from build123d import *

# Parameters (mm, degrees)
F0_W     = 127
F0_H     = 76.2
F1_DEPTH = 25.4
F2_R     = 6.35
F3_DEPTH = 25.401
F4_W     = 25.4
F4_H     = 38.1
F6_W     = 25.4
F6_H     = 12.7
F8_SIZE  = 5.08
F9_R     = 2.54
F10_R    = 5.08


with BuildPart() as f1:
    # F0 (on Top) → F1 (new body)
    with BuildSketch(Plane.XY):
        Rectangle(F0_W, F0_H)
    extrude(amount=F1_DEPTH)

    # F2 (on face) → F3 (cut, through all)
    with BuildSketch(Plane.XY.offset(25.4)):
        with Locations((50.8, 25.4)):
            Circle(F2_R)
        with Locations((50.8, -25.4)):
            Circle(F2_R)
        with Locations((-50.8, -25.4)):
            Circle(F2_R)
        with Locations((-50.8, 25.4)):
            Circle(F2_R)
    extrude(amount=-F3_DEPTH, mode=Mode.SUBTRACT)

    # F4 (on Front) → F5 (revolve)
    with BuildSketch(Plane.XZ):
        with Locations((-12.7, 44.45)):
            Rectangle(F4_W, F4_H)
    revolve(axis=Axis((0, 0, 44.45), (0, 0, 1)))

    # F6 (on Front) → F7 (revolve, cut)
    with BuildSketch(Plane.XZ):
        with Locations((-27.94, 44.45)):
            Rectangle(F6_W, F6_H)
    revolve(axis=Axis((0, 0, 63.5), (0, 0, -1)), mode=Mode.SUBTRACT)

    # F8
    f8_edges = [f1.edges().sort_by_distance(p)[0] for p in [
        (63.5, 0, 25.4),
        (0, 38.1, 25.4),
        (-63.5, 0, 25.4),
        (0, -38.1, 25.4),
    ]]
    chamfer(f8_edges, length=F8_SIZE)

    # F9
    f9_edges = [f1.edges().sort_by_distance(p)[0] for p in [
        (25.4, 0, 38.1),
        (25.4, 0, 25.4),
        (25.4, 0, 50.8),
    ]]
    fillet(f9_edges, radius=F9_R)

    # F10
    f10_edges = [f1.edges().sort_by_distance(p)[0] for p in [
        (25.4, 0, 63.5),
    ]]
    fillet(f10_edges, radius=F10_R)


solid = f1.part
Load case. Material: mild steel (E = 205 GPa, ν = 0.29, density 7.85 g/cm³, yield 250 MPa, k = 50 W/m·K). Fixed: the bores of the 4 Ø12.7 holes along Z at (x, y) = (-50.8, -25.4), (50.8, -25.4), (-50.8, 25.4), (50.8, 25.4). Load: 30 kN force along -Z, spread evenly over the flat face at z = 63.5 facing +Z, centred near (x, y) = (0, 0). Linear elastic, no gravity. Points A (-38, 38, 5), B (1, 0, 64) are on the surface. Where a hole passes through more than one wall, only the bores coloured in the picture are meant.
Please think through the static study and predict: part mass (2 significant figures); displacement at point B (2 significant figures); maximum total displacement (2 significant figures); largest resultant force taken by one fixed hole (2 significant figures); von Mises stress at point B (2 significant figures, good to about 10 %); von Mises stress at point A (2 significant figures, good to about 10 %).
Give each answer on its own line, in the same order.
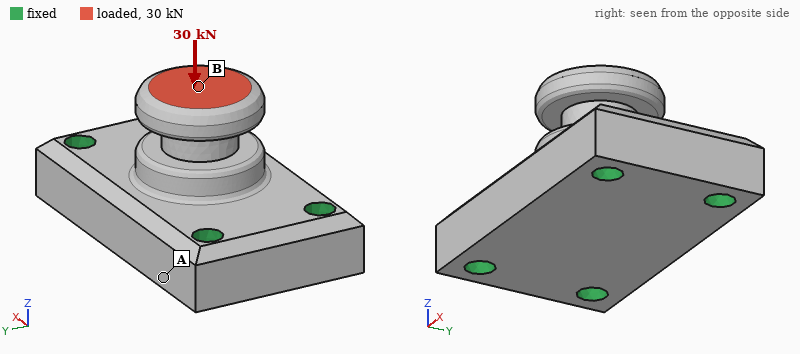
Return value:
2.3 kg
14 µm
15 µm
7.8 kN
39 MPa
11 MPa
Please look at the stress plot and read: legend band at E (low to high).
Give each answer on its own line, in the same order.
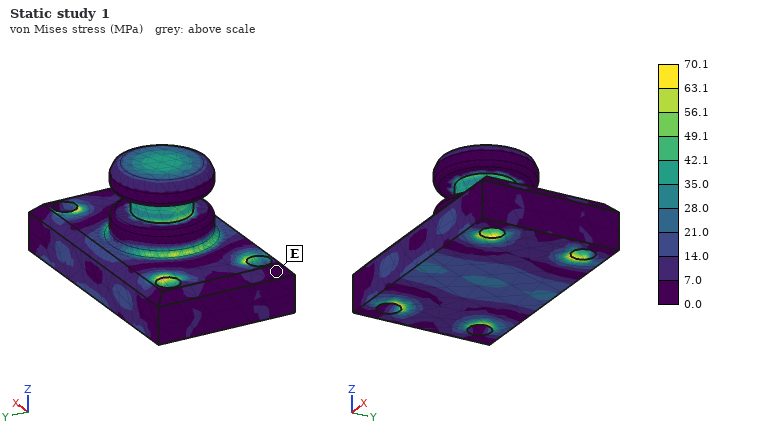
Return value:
0.0 to 7.0 MPa
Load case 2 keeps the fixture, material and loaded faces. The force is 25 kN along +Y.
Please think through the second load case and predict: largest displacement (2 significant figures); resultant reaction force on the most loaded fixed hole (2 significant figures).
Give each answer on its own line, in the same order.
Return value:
85 µm
14 kN
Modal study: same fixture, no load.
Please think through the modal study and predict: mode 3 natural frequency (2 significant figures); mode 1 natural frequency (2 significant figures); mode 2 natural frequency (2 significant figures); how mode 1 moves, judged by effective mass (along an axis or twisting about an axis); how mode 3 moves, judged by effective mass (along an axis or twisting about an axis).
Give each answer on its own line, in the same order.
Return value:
8400 Hz
6500 Hz
8100 Hz
along Y
along Z
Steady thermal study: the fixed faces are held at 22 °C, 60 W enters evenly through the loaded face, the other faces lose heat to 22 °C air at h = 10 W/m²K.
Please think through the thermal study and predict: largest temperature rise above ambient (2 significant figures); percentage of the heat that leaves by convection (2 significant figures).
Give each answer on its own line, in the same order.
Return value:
60 K
6.7 %
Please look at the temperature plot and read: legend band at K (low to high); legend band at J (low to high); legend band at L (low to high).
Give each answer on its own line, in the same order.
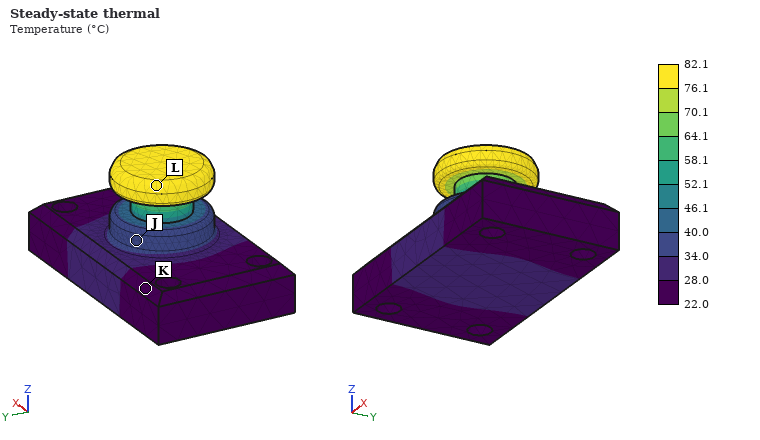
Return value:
22.0 to 28.0 °C
34.0 to 40.0 °C
76.1 to 82.1 °C
